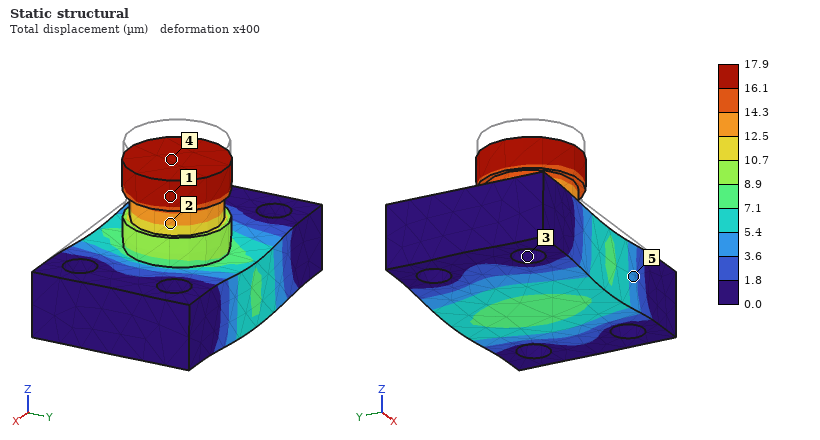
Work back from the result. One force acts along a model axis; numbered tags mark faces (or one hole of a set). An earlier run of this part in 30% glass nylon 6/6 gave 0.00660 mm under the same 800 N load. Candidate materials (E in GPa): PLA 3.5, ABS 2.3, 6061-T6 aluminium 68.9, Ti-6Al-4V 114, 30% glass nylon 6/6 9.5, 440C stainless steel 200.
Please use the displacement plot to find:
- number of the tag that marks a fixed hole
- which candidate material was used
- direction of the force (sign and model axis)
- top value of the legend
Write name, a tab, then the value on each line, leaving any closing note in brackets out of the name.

number of the tag that marks a fixed hole	3
which candidate material was used	PLA
direction of the force	-Z
top value of the legend	17.9 µm
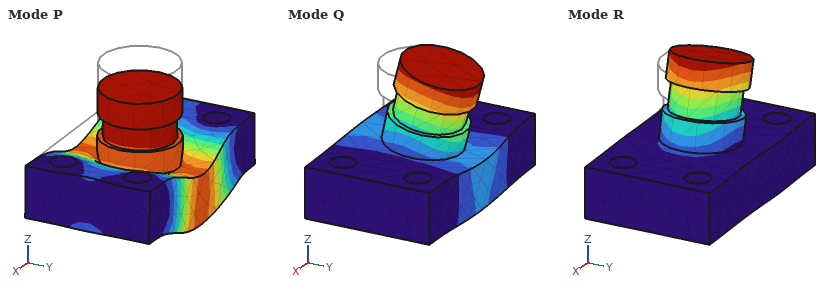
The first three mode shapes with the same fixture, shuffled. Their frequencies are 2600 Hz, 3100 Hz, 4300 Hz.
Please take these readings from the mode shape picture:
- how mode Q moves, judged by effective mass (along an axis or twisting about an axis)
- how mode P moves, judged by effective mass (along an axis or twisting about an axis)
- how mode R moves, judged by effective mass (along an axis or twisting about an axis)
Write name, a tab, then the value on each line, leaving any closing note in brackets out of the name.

how mode Q moves, judged by effective mass	along Y
how mode P moves, judged by effective mass	along Z
how mode R moves, judged by effective mass	along X
